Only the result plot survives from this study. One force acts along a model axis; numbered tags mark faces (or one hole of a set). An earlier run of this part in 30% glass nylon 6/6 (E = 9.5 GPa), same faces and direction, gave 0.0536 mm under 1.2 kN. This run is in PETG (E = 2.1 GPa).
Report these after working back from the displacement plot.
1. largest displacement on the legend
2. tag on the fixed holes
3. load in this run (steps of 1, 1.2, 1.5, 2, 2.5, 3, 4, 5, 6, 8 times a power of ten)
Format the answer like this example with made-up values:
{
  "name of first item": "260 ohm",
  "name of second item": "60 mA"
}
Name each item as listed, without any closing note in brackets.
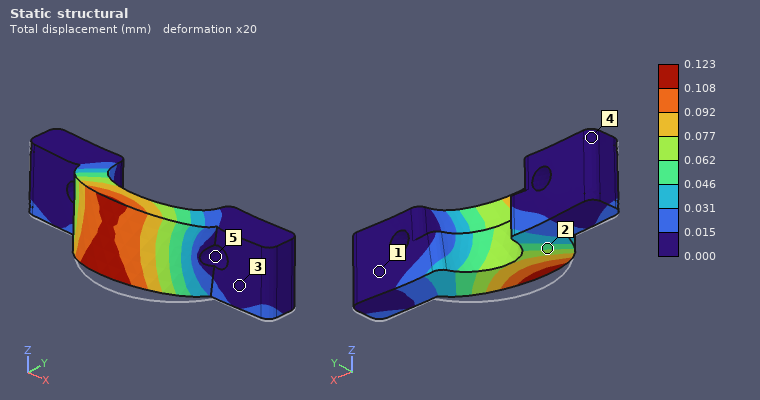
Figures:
{
  "largest displacement on the legend": "0.123 mm",
  "tag on the fixed holes": "5",
  "load in this run": "600 N"
}
